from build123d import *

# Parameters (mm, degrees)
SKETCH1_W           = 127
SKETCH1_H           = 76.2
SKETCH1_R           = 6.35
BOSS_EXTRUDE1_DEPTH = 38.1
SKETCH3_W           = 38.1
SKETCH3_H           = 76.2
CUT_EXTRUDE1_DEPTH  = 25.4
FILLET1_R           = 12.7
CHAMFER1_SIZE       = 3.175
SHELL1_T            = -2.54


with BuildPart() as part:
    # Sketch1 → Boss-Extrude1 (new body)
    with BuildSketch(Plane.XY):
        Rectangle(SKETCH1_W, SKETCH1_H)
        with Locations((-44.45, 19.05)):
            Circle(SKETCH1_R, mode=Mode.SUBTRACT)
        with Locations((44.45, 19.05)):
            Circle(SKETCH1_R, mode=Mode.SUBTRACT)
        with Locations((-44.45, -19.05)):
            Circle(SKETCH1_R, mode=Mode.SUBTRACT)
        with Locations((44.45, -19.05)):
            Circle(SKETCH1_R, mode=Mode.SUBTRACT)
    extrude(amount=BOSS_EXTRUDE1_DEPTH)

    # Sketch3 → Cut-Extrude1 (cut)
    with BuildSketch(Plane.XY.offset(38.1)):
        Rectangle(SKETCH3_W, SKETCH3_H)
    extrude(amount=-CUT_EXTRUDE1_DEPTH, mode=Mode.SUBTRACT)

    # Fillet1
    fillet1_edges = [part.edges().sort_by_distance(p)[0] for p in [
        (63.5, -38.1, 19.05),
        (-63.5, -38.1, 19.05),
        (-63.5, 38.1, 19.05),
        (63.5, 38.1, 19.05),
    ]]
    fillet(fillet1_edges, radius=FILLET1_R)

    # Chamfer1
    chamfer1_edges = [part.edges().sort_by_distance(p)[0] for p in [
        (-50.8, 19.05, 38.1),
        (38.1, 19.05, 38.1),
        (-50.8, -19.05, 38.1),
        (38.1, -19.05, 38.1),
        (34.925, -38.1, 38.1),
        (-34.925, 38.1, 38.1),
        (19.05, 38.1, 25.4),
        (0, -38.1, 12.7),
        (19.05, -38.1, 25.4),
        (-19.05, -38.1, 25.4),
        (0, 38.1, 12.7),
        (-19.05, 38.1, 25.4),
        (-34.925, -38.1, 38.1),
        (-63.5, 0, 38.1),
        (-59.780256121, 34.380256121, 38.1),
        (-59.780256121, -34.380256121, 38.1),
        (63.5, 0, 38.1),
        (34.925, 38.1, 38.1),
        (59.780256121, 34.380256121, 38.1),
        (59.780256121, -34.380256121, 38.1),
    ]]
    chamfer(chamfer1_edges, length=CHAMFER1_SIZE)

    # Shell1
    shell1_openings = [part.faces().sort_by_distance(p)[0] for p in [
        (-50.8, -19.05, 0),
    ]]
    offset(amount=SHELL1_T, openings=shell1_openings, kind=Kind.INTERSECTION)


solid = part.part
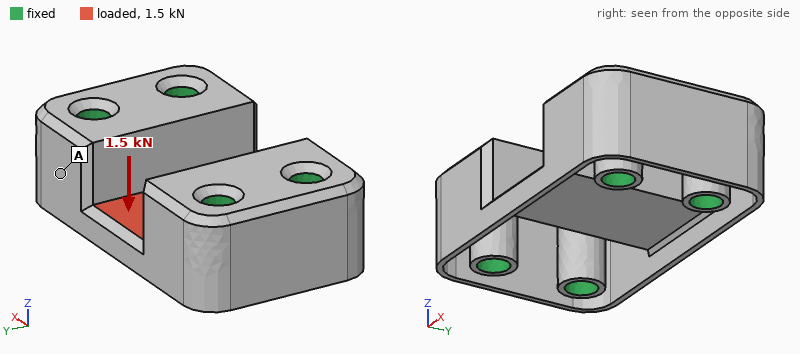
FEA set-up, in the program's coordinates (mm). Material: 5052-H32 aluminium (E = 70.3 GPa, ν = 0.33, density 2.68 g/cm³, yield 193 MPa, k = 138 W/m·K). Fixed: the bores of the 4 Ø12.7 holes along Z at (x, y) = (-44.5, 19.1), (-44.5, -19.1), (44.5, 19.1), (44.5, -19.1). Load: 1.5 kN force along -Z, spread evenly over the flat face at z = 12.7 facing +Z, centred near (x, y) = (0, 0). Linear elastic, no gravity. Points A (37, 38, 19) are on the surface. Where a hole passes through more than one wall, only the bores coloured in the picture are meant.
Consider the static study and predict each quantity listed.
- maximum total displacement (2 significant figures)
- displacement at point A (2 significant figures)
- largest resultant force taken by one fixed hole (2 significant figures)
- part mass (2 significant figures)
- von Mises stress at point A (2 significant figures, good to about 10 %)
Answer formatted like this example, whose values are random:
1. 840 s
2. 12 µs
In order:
1. 85 µm
2. 17 µm
3. 520 N
4. 200 g
5. 5.9 MPa
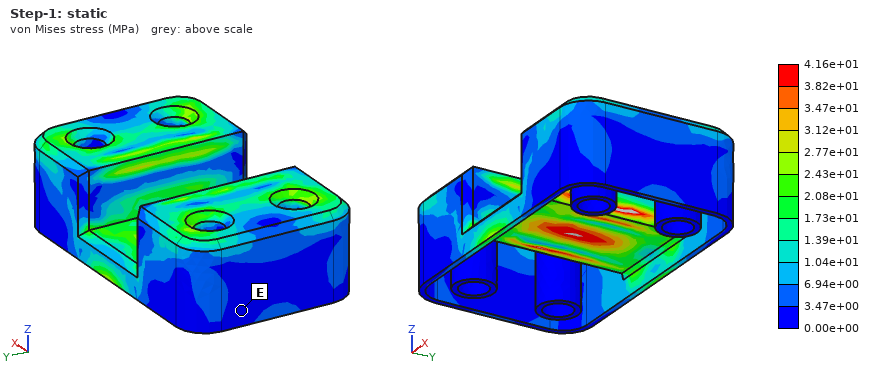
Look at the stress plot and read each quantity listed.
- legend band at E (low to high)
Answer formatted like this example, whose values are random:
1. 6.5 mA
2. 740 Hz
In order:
1. 0.00e+00 to 3.47e+00 MPa
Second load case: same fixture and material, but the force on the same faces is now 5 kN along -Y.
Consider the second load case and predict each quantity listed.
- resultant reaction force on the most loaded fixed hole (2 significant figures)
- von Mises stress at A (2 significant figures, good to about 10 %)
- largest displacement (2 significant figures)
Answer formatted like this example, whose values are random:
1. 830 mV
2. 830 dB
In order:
1. 2.5 kN
2. 26 MPa
3. 0.16 mm
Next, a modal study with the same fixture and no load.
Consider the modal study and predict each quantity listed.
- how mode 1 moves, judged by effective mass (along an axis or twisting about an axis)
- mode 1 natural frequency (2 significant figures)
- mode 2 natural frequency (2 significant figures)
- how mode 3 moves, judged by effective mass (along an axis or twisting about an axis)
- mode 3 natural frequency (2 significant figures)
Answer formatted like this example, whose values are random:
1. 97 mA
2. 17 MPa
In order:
1. along X
2. 2700 Hz
3. 2900 Hz
4. along Y
5. 3200 Hz
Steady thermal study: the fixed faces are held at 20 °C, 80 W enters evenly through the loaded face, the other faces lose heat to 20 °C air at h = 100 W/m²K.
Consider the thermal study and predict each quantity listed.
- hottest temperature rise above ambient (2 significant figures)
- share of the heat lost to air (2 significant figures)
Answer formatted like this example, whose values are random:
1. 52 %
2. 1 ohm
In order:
1. 42 K
2. 58 %
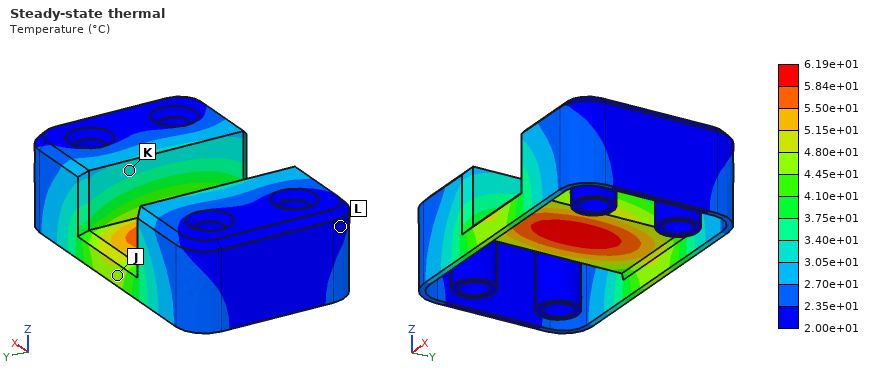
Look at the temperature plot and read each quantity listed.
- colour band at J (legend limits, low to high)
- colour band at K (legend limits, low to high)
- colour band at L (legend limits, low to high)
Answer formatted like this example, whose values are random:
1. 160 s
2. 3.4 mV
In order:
1. 4.45e+01 to 4.80e+01 °C
2. 3.05e+01 to 3.40e+01 °C
3. 2.00e+01 to 2.35e+01 °C
